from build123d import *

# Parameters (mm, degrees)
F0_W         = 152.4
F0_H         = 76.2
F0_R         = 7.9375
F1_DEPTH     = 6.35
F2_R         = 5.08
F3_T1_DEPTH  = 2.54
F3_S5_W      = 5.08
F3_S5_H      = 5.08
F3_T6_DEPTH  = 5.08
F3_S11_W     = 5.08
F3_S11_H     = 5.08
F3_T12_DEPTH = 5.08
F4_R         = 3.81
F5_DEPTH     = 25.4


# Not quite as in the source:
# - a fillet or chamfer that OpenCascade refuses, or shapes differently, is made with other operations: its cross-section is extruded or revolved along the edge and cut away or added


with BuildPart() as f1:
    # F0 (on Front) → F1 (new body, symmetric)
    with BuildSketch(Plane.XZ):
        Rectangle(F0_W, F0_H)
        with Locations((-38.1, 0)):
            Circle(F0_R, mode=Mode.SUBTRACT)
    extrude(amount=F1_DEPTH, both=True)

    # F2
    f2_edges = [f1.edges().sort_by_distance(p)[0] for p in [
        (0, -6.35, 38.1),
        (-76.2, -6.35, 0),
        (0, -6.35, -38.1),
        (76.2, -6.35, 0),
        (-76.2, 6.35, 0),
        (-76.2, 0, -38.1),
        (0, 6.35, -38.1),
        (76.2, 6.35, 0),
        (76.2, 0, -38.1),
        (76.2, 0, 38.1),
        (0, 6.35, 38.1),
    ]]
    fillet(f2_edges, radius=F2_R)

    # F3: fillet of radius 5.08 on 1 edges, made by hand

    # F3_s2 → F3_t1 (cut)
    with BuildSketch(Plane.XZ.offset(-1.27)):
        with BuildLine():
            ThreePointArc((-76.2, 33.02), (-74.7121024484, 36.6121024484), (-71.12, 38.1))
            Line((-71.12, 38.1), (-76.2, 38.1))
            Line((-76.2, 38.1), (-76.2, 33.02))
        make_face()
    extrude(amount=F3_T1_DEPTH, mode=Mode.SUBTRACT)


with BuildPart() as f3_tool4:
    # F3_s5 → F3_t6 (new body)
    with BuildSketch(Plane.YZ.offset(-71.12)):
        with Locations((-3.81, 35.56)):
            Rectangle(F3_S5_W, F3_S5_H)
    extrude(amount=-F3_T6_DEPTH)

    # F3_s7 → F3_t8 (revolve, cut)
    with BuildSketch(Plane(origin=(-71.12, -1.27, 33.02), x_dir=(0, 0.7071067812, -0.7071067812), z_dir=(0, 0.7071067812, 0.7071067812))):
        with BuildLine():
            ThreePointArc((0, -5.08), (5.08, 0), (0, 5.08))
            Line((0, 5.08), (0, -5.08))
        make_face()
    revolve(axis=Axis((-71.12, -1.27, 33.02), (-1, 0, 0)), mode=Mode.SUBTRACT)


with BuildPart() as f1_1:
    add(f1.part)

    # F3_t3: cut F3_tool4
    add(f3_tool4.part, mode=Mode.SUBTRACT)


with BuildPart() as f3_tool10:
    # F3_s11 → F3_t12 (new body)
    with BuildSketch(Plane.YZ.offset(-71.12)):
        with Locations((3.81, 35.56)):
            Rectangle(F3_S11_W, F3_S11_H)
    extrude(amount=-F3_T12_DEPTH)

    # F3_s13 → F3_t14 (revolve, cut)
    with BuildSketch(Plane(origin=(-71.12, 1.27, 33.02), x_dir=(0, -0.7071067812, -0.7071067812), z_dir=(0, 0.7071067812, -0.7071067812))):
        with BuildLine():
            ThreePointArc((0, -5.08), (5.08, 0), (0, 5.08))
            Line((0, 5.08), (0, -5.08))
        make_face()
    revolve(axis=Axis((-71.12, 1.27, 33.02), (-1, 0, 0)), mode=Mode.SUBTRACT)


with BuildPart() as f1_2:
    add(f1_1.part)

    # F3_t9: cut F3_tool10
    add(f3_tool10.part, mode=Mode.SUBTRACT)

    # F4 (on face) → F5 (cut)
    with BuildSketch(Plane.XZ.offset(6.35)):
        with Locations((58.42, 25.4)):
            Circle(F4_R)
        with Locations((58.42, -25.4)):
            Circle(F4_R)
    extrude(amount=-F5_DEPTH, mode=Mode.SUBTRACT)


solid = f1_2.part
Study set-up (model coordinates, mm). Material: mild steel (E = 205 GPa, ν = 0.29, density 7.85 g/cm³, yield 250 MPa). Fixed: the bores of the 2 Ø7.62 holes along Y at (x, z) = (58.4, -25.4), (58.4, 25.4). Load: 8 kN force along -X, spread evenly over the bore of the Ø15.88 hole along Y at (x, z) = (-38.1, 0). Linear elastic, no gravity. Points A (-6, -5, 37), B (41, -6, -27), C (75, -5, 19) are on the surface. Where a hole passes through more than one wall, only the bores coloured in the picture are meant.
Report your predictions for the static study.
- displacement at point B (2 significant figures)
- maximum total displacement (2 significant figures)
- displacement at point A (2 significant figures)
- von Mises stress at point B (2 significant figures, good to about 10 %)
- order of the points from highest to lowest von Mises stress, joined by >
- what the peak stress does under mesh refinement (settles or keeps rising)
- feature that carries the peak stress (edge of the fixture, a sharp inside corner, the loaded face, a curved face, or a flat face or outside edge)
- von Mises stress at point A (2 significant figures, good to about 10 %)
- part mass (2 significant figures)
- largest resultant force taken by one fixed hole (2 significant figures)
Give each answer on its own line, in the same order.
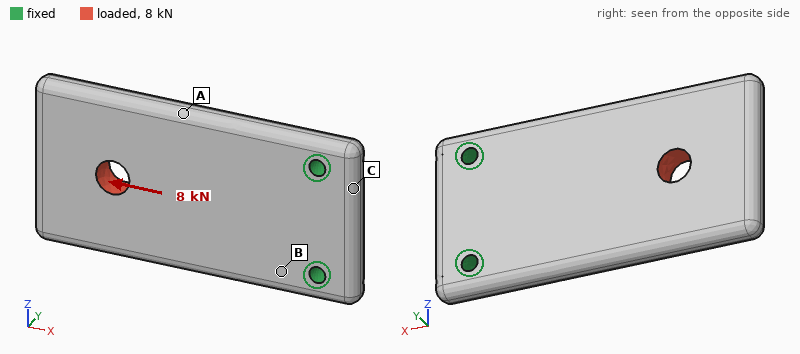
0.97 µm
5.8 µm
3.0 µm
11 MPa
B > A > C
keeps rising
edge of the fixture
7.0 MPa
1.1 kg
4.0 kN
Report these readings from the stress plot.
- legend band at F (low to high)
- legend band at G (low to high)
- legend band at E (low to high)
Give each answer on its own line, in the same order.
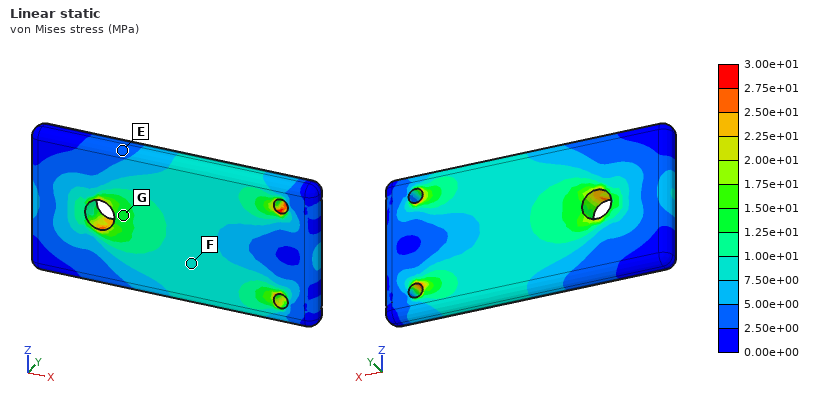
7.50e+00 to 1.00e+01 MPa
1.25e+01 to 1.50e+01 MPa
2.50e+00 to 5.00e+00 MPa
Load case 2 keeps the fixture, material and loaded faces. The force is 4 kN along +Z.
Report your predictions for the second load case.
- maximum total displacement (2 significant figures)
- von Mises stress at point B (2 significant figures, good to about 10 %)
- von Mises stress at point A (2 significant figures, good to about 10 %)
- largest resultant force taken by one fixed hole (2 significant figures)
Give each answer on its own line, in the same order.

30 µm
22 MPa
11 MPa
7.4 kN
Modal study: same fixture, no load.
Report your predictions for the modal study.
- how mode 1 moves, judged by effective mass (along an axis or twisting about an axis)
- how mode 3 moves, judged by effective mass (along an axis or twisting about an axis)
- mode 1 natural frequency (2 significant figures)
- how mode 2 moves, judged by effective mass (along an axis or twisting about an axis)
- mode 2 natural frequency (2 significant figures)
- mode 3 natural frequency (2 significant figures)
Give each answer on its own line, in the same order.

along Y
along Z
570 Hz
twisting about X
2200 Hz
2800 Hz
